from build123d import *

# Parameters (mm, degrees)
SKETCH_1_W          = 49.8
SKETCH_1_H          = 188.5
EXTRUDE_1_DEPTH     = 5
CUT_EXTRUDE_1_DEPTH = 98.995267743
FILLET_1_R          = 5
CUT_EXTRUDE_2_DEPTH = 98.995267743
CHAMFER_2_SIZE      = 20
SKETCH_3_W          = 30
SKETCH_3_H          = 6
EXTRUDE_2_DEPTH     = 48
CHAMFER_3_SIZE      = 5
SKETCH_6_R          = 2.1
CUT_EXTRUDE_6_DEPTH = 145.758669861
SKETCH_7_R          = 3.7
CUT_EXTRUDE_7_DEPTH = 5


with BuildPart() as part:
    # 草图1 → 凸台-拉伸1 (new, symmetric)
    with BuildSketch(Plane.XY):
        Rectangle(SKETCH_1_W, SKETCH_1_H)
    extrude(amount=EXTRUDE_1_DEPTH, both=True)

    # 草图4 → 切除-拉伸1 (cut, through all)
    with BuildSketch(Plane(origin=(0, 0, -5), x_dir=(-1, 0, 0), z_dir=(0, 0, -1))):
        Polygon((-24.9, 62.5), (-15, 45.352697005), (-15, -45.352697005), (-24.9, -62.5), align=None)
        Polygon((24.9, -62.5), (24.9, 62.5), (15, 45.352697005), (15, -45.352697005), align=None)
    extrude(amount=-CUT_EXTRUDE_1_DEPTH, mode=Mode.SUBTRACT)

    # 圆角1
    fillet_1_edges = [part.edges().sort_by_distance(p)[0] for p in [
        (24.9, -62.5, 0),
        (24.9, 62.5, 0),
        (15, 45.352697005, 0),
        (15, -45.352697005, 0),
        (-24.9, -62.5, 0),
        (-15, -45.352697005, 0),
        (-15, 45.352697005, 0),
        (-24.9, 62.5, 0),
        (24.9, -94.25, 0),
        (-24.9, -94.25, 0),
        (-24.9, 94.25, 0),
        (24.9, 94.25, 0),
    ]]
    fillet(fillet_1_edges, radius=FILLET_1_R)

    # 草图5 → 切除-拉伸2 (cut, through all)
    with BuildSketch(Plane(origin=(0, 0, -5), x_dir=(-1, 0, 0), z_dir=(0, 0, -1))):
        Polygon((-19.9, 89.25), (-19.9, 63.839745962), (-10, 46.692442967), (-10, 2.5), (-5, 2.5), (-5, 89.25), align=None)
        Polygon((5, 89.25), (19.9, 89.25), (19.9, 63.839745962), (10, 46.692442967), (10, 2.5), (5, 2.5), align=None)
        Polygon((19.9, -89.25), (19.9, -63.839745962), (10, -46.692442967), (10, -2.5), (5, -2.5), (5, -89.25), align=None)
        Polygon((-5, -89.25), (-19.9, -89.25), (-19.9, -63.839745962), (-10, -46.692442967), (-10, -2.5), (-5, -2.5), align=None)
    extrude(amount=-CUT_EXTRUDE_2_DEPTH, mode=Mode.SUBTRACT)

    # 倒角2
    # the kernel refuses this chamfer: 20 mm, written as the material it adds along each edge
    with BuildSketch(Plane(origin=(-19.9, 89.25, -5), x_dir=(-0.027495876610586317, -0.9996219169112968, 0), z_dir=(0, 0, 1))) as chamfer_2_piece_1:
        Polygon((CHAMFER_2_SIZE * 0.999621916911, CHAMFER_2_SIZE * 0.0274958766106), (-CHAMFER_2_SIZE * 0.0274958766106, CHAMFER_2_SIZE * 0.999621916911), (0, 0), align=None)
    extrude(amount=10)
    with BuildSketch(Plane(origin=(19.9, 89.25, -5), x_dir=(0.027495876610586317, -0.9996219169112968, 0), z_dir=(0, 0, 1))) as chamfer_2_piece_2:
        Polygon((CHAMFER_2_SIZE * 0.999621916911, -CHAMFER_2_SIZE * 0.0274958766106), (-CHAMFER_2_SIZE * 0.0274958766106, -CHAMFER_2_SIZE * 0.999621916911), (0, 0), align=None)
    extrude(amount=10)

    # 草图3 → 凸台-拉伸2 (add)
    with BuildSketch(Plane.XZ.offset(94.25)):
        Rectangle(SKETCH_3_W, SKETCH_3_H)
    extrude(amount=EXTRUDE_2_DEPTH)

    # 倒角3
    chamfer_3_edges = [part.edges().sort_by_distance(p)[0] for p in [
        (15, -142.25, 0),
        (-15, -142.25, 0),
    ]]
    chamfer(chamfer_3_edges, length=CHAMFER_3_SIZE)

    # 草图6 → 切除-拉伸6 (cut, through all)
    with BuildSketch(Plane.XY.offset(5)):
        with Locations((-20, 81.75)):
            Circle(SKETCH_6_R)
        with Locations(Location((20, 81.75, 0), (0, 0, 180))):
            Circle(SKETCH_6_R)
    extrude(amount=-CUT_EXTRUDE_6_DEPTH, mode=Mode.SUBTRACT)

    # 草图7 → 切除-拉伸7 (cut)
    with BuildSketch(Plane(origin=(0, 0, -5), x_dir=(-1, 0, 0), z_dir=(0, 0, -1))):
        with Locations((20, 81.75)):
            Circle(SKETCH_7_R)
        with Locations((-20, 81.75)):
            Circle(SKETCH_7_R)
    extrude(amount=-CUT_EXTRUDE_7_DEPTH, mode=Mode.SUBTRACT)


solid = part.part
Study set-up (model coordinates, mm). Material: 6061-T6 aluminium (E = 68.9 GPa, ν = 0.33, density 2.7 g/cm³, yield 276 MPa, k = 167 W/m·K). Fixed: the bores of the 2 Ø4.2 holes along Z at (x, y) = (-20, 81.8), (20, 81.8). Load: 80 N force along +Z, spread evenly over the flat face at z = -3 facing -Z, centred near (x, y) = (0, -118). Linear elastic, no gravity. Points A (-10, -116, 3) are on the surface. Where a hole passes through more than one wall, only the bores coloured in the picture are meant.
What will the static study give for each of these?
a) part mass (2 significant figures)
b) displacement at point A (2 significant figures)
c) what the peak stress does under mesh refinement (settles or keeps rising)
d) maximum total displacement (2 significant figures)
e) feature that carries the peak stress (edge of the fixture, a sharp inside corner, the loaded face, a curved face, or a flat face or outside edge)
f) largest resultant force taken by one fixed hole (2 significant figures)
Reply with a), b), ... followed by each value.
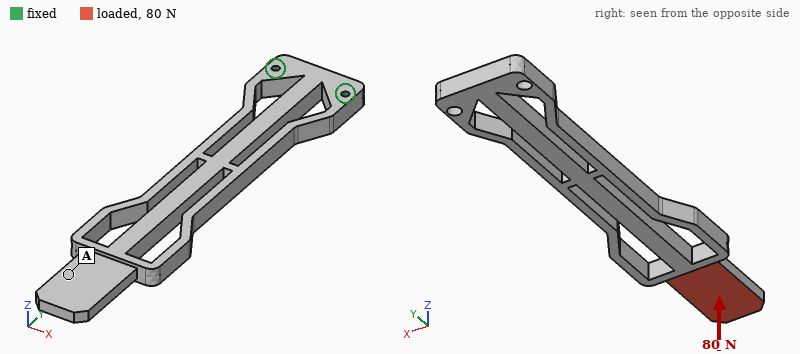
a) 140 g
b) 2.3 mm
c) keeps rising
d) 2.7 mm
e) edge of the fixture
f) 40 N
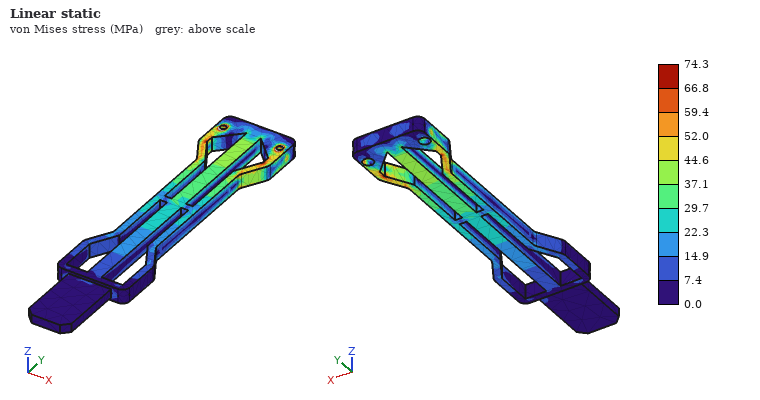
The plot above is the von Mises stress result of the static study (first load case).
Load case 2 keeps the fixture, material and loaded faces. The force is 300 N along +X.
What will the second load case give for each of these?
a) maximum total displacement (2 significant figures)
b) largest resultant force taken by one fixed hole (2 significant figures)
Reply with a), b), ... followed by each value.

a) 2.3 mm
b) 1.4 kN
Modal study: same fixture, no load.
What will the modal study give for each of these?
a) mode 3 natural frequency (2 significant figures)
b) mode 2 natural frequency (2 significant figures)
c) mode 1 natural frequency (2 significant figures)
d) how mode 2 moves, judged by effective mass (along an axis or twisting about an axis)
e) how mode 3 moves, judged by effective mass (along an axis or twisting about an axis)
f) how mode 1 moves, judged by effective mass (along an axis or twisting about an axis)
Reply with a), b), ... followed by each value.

a) 890 Hz
b) 320 Hz
c) 140 Hz
d) along X
e) along Z
f) along Z
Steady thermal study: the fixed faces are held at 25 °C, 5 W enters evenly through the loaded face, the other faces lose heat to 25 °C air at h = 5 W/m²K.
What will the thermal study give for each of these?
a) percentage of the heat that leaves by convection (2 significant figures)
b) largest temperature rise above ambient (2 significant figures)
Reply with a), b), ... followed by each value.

a) 26 %
b) 26 K
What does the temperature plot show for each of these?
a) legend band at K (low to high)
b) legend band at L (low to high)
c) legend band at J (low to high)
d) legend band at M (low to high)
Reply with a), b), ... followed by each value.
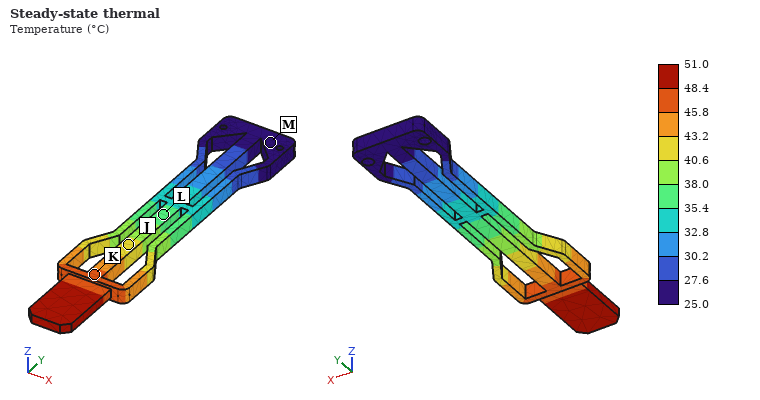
a) 45.8 to 48.4 °C
b) 35.4 to 38.0 °C
c) 40.6 to 43.2 °C
d) 25.0 to 27.6 °C
